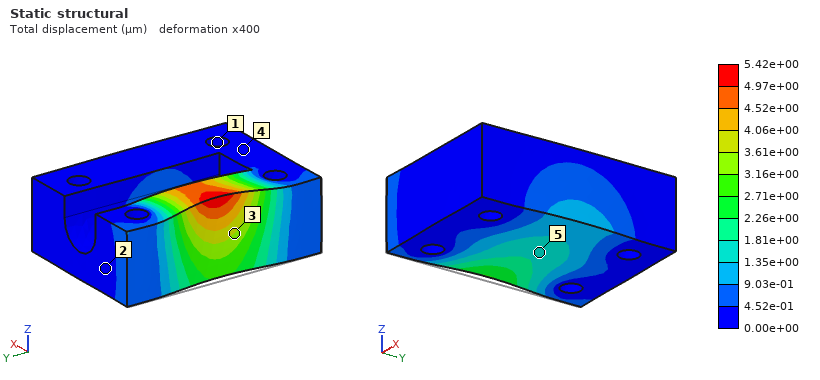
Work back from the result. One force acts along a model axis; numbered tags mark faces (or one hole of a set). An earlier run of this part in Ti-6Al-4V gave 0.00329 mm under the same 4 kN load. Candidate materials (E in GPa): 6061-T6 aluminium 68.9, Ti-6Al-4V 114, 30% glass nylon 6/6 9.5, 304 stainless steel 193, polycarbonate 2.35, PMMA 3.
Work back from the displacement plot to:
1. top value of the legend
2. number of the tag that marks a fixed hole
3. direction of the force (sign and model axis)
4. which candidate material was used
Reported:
5.42e+00 µm
1
+X
6061-T6 aluminium
